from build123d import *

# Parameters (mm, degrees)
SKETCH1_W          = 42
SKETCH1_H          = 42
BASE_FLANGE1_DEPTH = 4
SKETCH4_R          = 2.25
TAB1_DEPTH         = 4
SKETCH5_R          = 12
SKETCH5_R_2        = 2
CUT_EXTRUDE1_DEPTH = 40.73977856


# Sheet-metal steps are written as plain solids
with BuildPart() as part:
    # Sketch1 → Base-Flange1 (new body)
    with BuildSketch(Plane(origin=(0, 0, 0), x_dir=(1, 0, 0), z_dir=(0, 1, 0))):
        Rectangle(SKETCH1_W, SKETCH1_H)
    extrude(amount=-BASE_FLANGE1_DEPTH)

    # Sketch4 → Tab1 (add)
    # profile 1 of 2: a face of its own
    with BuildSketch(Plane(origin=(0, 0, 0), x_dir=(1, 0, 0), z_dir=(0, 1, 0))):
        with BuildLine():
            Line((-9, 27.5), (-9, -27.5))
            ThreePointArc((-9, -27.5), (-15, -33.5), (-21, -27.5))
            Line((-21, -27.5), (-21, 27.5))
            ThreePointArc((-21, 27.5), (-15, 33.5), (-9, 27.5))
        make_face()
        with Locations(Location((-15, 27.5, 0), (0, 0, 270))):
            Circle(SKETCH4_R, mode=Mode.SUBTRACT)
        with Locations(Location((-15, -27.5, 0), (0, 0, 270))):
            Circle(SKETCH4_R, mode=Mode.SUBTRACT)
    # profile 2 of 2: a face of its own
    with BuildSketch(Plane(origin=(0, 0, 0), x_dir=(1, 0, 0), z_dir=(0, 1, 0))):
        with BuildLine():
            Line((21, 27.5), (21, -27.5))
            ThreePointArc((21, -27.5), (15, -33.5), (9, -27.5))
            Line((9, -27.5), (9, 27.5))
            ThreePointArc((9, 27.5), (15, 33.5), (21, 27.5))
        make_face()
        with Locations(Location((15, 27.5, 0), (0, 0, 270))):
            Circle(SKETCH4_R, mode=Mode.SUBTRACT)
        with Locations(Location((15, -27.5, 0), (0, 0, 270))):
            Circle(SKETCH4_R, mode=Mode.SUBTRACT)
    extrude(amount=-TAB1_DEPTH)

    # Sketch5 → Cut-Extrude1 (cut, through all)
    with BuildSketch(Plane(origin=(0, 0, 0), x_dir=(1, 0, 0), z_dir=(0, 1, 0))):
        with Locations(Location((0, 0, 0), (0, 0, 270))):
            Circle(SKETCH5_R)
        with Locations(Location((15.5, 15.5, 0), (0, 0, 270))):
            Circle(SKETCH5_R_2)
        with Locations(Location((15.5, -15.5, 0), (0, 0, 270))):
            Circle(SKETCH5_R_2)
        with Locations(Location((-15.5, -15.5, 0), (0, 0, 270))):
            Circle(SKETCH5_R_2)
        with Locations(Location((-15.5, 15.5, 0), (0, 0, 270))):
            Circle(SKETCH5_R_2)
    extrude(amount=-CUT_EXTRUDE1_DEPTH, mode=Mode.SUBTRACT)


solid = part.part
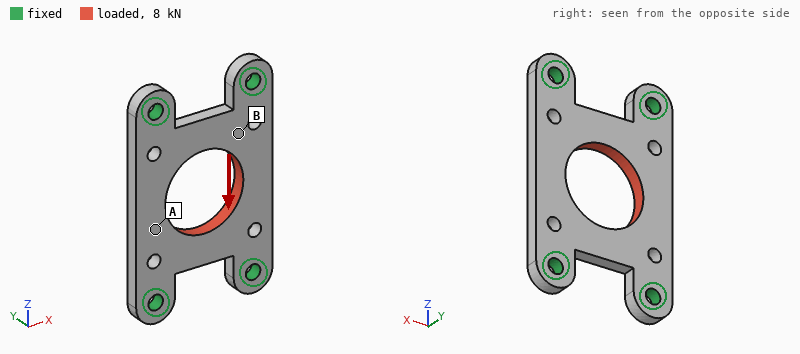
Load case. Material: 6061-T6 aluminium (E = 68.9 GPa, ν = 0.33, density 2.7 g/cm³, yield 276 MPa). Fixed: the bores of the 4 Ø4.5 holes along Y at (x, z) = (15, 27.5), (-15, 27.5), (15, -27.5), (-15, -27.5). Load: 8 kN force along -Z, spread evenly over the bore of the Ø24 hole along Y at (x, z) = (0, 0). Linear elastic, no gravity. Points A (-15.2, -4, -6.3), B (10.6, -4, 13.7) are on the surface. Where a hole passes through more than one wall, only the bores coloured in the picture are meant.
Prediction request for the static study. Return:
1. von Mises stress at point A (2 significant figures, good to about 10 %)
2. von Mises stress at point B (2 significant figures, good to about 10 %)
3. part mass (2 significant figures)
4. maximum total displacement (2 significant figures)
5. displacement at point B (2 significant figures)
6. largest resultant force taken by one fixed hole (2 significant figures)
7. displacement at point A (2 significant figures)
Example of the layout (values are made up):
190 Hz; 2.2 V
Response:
24 MPa; 45 MPa; 19 g; 18 µm; 10 µm; 2.1 kN; 11 µm
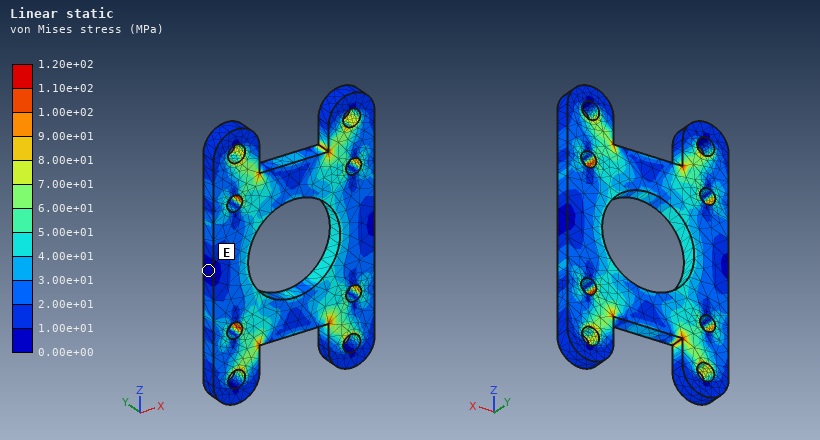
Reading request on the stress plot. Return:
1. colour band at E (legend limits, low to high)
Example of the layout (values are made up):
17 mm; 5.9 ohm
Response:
0.00e+00 to 1.00e+01 MPa
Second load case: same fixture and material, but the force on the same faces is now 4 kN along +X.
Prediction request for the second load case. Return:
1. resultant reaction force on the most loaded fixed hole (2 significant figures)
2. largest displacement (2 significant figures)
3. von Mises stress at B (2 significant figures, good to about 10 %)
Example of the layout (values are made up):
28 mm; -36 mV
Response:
1.1 kN; 30 µm; 17 MPa
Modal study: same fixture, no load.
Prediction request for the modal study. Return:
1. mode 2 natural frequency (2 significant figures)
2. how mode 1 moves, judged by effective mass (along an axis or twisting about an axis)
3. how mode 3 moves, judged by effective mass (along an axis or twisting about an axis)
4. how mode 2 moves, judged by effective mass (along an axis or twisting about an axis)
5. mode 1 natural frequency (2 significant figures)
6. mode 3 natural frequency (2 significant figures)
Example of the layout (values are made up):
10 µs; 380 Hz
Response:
8500 Hz; along Y; twisting about X; twisting about Z; 6900 Hz; 14 kHz
